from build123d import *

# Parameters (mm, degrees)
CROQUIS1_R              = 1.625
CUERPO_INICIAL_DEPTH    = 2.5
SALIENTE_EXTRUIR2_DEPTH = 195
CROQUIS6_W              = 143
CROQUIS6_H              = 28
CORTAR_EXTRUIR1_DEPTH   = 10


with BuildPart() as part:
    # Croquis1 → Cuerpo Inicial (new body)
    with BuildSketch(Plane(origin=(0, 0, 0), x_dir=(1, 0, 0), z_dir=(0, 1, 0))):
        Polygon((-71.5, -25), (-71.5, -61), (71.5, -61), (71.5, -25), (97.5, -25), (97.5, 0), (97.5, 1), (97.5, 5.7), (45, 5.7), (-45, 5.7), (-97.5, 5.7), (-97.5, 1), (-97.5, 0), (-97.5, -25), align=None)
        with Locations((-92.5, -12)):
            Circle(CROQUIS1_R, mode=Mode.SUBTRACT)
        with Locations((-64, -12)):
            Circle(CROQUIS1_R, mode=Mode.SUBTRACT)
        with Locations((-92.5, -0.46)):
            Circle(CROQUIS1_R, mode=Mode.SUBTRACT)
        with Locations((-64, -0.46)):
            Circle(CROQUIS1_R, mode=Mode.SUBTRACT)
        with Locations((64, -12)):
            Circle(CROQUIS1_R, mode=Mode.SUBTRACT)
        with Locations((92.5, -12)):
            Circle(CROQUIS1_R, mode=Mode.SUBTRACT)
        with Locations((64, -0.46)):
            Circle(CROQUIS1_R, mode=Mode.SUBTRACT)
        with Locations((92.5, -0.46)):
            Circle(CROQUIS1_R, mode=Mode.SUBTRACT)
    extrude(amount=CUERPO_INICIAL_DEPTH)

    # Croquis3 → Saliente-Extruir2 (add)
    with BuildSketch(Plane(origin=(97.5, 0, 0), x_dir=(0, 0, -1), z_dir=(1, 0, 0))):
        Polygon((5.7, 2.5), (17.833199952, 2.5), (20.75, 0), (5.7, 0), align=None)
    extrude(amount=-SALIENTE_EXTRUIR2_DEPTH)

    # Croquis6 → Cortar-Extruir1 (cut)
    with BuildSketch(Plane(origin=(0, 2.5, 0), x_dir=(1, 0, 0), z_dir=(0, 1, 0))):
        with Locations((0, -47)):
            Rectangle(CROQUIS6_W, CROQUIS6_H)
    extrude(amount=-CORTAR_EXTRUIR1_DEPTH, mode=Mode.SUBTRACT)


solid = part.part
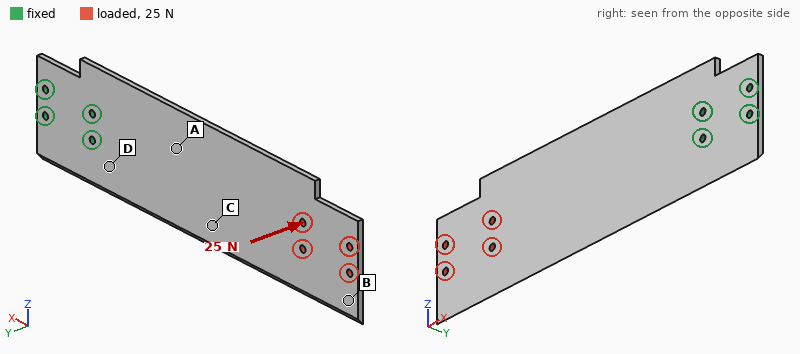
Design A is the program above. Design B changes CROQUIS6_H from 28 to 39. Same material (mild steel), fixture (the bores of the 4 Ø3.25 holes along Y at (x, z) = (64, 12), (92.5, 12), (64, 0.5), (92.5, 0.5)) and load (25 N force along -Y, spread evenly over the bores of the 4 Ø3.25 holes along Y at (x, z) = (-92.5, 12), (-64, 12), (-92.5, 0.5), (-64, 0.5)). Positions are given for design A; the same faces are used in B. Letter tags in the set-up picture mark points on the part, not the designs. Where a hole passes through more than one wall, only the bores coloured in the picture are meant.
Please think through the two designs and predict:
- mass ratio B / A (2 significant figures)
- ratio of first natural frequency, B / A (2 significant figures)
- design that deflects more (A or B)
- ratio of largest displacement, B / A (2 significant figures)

0.92
0.98
B
1.1
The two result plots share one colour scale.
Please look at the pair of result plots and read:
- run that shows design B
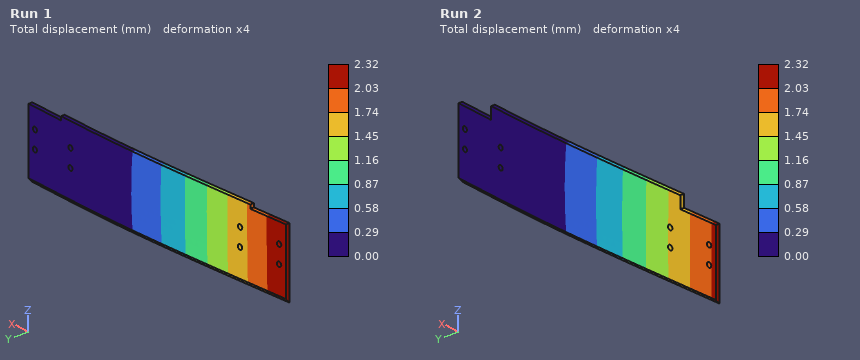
Run 1
